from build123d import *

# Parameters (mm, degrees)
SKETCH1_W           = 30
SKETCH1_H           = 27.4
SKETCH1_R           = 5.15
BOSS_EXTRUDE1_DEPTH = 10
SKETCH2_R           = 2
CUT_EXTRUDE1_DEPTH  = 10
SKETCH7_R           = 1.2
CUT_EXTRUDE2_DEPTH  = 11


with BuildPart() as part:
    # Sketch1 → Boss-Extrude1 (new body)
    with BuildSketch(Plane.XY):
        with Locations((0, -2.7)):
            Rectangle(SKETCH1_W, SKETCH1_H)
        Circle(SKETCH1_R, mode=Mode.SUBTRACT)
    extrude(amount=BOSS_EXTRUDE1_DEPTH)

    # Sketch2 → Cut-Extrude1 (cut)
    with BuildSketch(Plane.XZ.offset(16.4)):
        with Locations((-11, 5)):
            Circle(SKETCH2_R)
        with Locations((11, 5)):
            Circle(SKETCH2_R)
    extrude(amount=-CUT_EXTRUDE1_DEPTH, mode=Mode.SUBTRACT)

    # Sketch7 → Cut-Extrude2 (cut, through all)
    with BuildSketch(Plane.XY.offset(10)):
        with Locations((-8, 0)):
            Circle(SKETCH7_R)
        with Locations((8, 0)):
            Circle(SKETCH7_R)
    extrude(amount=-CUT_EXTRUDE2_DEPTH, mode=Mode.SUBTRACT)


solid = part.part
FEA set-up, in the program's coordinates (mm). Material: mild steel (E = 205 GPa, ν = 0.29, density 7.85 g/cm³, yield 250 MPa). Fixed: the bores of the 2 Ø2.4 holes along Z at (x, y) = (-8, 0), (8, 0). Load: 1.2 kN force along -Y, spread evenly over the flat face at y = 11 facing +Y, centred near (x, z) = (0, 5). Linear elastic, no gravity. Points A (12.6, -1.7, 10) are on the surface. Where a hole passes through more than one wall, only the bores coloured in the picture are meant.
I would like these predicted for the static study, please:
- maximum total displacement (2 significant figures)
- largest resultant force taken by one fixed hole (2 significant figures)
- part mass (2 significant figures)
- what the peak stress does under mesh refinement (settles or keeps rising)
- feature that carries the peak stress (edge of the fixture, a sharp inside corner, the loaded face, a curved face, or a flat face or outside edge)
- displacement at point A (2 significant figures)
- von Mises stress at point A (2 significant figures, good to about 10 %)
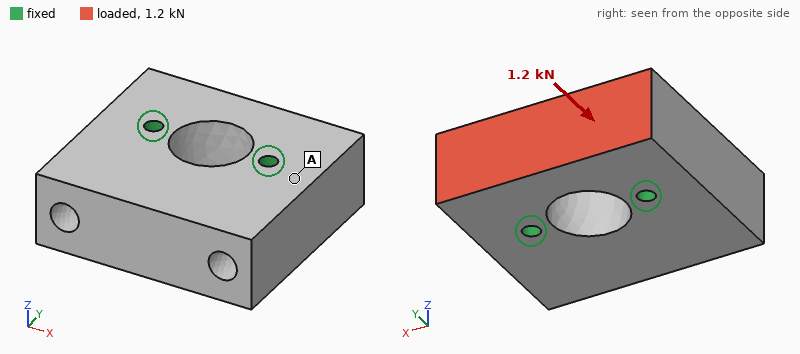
0.44 µm
610 N
55 g
keeps rising
edge of the fixture
0.11 µm
2.2 MPa
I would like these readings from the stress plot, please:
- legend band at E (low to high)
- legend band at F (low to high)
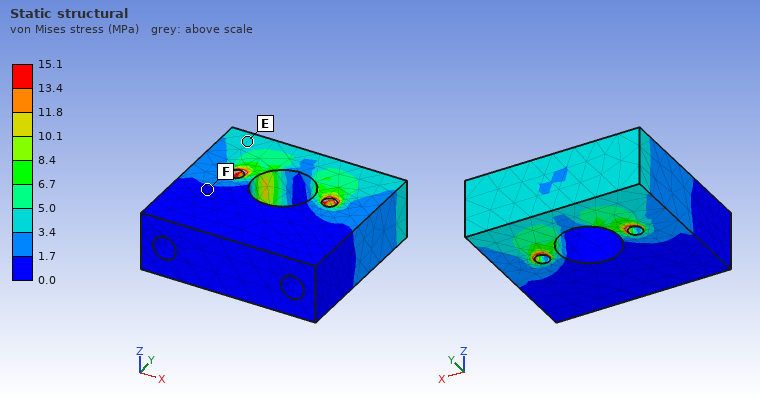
3.4 to 5.0 MPa
0.0 to 1.7 MPa
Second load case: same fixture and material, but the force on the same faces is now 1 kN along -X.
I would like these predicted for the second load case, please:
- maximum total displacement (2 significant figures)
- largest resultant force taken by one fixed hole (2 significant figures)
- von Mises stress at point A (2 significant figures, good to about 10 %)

1.8 µm
730 N
4.4 MPa
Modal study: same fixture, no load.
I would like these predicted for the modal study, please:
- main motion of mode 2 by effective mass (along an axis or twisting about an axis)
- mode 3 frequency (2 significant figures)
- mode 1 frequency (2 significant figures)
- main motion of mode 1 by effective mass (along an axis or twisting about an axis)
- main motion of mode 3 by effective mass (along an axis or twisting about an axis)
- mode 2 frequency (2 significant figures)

along X
30 kHz
20 kHz
along Z
twisting about Y
27 kHz
